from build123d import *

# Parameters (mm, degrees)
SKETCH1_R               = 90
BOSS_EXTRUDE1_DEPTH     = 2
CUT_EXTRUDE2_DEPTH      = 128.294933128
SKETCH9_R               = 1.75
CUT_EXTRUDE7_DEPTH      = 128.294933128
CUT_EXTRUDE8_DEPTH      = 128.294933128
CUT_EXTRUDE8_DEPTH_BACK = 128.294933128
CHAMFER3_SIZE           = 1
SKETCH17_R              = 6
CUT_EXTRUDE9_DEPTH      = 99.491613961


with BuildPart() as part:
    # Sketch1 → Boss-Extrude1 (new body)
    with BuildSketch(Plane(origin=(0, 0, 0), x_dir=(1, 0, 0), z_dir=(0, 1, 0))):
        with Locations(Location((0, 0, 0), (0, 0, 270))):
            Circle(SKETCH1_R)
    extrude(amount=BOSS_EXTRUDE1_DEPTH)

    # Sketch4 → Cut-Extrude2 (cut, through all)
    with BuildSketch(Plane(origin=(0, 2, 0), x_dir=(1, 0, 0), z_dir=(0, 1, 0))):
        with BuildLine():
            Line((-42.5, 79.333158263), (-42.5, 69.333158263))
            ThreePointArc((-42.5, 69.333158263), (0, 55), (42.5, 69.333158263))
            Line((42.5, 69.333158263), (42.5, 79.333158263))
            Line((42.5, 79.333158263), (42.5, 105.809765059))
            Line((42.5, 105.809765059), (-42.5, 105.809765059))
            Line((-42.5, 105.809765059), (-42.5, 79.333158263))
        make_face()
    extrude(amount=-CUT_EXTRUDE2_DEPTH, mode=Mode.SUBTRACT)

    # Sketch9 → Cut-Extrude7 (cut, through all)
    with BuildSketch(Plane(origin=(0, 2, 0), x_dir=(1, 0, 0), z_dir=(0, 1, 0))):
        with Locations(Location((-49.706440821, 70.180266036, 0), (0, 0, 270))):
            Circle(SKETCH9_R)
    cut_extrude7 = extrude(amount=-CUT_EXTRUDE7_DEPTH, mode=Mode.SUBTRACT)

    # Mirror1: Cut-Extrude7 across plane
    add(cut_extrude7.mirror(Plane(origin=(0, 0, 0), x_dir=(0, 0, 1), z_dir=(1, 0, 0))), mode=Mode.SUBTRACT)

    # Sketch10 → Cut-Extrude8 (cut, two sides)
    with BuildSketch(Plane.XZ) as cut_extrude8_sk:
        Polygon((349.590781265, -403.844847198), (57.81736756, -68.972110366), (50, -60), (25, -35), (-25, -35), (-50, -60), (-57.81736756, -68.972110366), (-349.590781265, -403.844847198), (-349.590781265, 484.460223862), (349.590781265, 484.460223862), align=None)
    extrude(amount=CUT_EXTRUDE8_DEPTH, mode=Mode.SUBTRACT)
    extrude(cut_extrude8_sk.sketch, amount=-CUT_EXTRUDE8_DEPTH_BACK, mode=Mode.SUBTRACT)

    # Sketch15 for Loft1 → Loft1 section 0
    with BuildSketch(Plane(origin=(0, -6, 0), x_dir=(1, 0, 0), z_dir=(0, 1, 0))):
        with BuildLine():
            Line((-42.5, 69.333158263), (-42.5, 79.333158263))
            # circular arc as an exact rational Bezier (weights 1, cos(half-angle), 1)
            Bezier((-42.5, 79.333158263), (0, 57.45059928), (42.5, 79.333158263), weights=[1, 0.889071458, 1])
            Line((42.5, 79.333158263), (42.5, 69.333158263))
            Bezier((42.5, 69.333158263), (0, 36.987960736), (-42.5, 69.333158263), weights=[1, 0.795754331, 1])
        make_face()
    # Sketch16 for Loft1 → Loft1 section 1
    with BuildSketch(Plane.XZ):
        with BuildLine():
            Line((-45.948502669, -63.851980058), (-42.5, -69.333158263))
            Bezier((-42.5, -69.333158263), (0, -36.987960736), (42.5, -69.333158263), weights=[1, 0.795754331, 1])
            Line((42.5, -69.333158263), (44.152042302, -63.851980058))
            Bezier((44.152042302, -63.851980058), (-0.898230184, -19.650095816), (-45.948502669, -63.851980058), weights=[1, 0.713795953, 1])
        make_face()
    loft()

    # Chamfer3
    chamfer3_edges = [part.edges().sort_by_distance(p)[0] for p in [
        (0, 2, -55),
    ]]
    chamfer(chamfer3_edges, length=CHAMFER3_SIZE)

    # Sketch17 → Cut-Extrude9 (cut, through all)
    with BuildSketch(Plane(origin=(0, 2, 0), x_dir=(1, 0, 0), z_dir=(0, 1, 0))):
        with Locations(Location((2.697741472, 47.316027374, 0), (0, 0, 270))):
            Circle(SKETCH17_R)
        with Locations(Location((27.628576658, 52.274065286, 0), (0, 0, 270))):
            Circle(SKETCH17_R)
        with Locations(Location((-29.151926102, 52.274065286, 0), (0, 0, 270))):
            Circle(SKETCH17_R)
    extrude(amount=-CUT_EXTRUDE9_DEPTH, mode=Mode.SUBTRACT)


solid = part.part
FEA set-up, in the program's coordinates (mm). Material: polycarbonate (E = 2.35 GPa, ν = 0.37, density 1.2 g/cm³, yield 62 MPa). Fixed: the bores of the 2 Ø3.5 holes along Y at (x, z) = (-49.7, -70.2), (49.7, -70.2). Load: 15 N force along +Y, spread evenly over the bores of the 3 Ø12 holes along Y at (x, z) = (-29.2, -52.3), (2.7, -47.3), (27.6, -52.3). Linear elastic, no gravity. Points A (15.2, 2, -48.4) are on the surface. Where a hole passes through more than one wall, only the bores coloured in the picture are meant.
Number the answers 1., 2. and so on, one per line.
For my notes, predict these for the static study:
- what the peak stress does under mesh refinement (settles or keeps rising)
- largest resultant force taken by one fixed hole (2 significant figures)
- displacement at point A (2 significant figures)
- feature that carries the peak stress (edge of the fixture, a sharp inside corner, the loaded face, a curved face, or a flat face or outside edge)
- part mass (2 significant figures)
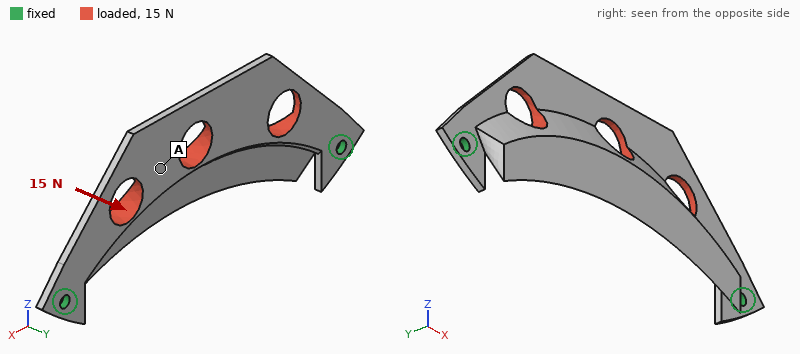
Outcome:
1. keeps rising
2. 22 N
3. 0.82 mm
4. edge of the fixture
5. 11 g
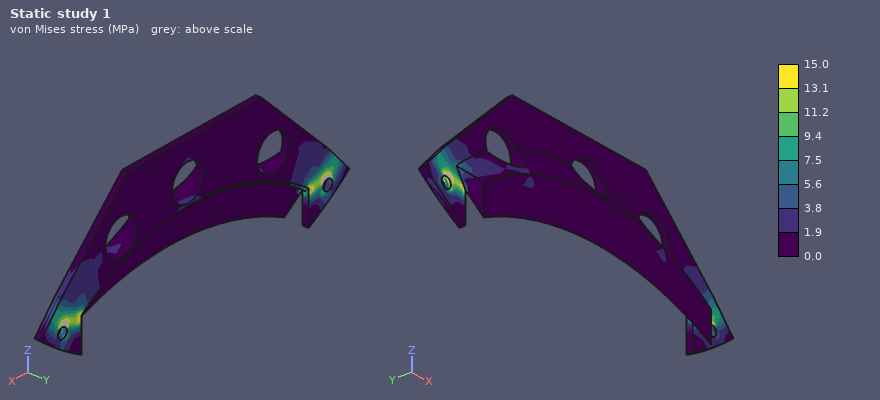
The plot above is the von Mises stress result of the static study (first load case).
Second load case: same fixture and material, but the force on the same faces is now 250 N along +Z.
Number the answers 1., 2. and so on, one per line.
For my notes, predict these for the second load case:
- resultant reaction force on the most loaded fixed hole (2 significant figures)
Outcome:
1. 170 N
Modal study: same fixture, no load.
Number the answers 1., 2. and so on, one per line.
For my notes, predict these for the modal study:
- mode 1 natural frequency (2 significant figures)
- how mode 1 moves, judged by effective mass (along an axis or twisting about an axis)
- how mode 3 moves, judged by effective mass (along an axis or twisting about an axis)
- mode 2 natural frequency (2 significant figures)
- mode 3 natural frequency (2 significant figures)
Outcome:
1. 260 Hz
2. along Y
3. along Y
4. 960 Hz
5. 1100 Hz
